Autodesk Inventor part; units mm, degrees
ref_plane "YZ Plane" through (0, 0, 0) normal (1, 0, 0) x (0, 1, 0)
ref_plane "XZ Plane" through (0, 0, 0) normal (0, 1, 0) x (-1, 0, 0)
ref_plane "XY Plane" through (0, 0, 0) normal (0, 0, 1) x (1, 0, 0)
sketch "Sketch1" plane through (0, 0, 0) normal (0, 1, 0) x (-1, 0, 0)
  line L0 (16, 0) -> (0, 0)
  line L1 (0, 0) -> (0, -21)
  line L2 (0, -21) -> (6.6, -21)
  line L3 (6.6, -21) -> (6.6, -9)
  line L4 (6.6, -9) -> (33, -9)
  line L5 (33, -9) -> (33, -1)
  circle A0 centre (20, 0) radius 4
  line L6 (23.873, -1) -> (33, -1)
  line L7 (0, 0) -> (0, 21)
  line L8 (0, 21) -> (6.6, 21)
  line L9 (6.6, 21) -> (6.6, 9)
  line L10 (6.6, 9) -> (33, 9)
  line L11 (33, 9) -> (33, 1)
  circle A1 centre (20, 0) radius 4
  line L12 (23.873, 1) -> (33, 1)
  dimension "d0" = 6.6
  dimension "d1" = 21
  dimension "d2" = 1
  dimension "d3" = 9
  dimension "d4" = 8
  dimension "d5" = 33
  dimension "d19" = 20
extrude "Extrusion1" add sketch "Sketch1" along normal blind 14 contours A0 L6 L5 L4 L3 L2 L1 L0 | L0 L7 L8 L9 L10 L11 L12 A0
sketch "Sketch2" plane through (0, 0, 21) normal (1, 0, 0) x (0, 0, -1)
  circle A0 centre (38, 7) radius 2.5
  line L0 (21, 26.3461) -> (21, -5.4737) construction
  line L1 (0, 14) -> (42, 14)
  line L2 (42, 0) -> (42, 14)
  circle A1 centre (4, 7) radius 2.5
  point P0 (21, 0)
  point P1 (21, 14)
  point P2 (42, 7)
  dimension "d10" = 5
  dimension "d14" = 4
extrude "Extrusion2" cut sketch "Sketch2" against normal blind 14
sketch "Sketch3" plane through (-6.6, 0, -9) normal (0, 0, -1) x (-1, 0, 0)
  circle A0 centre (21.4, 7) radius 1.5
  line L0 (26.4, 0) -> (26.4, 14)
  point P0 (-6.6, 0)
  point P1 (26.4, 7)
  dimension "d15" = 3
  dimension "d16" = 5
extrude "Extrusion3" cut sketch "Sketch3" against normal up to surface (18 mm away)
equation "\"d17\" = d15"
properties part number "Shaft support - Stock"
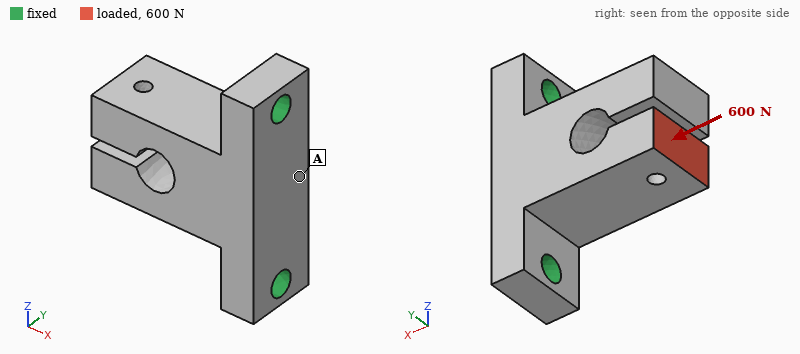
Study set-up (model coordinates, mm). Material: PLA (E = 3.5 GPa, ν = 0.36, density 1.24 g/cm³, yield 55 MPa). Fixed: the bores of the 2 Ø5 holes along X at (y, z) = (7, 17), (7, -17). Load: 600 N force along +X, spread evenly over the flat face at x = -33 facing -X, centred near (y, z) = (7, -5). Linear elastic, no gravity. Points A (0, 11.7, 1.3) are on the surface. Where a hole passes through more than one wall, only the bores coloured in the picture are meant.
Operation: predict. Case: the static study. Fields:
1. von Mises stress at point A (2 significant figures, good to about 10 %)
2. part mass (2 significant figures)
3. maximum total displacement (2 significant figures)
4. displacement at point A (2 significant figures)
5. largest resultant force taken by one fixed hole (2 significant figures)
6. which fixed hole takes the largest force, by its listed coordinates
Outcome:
3.7 MPa
11 g
0.17 mm
0.050 mm
430 N
(7, -17)
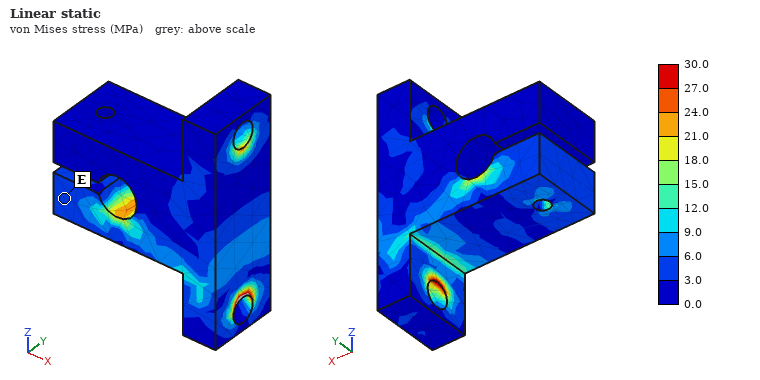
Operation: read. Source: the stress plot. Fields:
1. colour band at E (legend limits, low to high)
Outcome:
3.0 to 6.0 MPa
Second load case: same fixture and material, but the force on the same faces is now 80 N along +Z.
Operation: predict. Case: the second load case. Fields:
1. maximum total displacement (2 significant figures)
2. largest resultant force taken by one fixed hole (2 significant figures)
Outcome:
0.33 mm
110 N
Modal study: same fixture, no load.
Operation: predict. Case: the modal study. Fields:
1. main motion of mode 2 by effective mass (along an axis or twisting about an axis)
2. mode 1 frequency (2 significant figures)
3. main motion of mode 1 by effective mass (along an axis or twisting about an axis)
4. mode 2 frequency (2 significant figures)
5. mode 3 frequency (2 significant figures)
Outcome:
along Z
1700 Hz
along Y
2700 Hz
3300 Hz
